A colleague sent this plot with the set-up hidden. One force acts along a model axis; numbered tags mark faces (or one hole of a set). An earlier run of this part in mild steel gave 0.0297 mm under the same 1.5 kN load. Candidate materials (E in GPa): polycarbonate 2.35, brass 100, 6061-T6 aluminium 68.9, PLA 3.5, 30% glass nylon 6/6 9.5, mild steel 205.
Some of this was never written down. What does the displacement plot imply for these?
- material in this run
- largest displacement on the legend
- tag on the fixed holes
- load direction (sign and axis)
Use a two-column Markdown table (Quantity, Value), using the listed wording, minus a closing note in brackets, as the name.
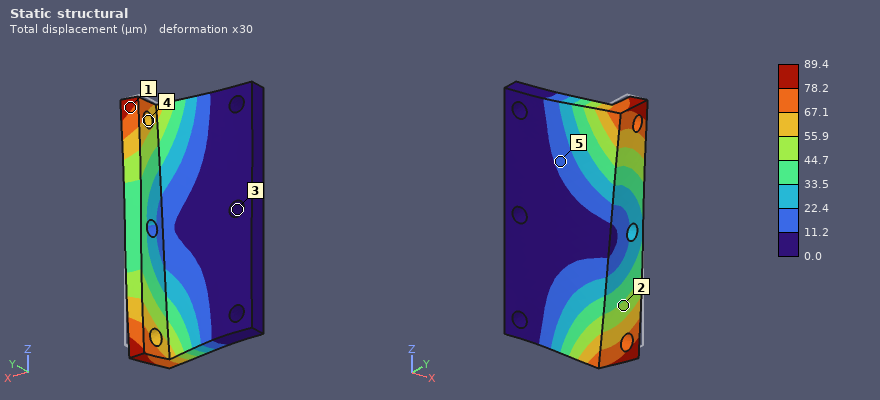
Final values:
| Quantity | Value |
|---|---|
| material in this run | 6061-T6 aluminium |
| largest displacement on the legend | 89.4 µm |
| tag on the fixed holes | 3 |
| load direction | -Z |
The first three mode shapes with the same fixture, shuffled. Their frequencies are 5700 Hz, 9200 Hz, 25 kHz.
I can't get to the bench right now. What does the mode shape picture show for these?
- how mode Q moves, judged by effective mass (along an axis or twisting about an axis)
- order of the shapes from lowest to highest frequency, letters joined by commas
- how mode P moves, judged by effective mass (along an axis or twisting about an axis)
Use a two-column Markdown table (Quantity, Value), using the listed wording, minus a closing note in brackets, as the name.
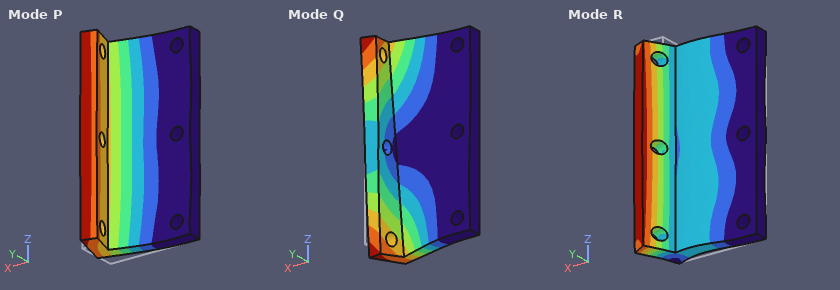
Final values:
| Quantity | Value |
|---|---|
| how mode Q moves, judged by effective mass | twisting about X |
| order of the shapes from lowest to highest frequency, letters joined by commas | P, Q, R |
| how mode P moves, judged by effective mass | along Y |
